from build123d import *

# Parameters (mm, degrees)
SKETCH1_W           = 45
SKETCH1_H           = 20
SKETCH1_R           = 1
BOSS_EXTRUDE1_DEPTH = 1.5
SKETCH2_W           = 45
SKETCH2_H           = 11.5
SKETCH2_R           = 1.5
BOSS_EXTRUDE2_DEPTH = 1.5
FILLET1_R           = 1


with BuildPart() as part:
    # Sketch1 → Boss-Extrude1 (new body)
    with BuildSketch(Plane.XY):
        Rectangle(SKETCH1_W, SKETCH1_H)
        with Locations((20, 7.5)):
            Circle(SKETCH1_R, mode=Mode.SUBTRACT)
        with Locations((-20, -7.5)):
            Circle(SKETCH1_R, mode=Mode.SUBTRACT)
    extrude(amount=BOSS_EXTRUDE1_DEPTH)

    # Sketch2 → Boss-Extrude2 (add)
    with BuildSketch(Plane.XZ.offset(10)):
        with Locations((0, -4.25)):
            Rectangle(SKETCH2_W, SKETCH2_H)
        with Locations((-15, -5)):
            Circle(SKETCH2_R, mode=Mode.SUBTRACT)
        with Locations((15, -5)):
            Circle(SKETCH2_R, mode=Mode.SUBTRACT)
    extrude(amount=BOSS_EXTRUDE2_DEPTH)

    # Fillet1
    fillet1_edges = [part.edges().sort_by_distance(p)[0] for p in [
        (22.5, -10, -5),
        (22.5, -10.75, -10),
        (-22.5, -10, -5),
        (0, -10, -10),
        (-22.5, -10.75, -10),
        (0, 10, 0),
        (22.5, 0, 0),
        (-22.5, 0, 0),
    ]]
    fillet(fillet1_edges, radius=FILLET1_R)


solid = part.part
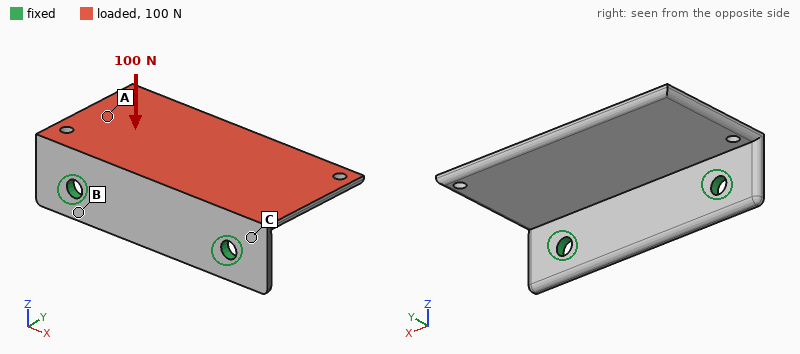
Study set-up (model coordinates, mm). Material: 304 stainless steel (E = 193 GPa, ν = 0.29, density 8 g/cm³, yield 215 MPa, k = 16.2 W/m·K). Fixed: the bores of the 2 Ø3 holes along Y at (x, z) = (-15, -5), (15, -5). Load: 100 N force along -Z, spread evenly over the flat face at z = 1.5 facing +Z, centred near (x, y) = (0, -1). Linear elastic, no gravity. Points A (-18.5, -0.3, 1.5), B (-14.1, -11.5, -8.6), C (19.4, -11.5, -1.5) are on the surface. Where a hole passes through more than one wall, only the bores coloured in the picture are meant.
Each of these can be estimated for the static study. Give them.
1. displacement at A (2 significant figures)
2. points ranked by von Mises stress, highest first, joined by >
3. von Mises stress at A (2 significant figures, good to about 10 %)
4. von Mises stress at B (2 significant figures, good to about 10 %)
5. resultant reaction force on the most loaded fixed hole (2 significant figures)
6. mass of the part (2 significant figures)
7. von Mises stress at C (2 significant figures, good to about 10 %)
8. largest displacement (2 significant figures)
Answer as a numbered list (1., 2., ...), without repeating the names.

1. 43 µm
2. C > B > A
3. 14 MPa
4. 36 MPa
5. 51 N
6. 17 g
7. 54 MPa
8. 96 µm
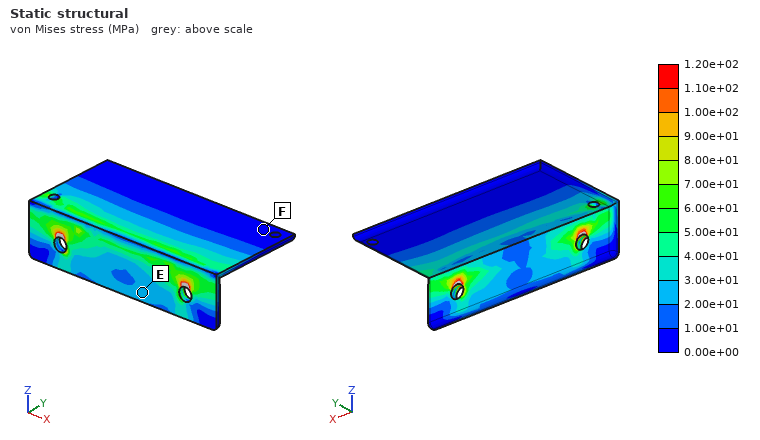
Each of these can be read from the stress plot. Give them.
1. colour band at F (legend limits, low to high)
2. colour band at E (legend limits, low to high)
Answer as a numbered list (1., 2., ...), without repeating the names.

1. 0.00e+00 to 1.00e+01 MPa
2. 2.00e+01 to 3.00e+01 MPa
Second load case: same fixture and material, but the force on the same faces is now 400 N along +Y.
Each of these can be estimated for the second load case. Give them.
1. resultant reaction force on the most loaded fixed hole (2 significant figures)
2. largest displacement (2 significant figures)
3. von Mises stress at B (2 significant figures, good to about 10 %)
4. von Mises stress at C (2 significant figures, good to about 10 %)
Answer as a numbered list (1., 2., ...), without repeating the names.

1. 200 N
2. 98 µm
3. 41 MPa
4. 75 MPa
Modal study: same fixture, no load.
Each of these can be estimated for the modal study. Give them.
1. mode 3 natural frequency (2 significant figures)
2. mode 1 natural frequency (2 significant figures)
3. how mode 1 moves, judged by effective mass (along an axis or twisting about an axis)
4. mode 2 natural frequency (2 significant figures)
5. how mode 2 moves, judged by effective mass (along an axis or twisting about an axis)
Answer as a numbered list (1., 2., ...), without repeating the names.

1. 7000 Hz
2. 1900 Hz
3. along Z
4. 3400 Hz
5. twisting about Y
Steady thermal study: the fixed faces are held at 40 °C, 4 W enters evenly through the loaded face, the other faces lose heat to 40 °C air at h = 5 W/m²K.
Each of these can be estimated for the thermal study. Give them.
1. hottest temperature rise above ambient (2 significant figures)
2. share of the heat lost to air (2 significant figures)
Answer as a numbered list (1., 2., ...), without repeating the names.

1. 65 K
2. 9.2 %
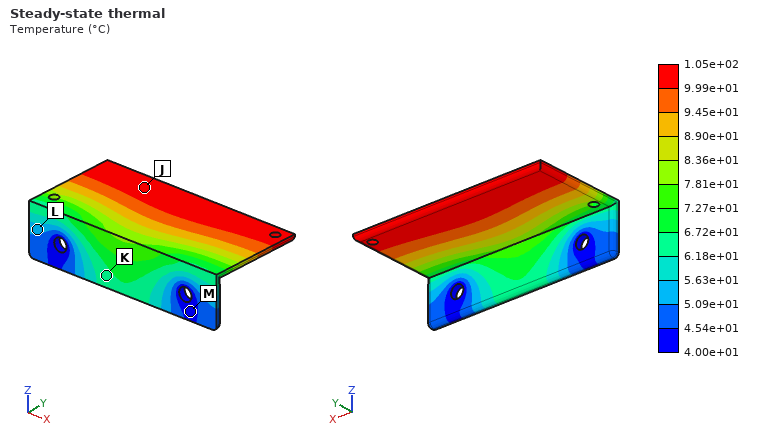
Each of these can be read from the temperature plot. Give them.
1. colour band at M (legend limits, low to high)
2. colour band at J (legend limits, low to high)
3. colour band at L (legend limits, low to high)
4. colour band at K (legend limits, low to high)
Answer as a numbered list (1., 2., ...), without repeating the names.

1. 4.00e+01 to 4.54e+01 °C
2. 9.99e+01 to 1.05e+02 °C
3. 5.09e+01 to 5.63e+01 °C
4. 6.18e+01 to 6.72e+01 °C
